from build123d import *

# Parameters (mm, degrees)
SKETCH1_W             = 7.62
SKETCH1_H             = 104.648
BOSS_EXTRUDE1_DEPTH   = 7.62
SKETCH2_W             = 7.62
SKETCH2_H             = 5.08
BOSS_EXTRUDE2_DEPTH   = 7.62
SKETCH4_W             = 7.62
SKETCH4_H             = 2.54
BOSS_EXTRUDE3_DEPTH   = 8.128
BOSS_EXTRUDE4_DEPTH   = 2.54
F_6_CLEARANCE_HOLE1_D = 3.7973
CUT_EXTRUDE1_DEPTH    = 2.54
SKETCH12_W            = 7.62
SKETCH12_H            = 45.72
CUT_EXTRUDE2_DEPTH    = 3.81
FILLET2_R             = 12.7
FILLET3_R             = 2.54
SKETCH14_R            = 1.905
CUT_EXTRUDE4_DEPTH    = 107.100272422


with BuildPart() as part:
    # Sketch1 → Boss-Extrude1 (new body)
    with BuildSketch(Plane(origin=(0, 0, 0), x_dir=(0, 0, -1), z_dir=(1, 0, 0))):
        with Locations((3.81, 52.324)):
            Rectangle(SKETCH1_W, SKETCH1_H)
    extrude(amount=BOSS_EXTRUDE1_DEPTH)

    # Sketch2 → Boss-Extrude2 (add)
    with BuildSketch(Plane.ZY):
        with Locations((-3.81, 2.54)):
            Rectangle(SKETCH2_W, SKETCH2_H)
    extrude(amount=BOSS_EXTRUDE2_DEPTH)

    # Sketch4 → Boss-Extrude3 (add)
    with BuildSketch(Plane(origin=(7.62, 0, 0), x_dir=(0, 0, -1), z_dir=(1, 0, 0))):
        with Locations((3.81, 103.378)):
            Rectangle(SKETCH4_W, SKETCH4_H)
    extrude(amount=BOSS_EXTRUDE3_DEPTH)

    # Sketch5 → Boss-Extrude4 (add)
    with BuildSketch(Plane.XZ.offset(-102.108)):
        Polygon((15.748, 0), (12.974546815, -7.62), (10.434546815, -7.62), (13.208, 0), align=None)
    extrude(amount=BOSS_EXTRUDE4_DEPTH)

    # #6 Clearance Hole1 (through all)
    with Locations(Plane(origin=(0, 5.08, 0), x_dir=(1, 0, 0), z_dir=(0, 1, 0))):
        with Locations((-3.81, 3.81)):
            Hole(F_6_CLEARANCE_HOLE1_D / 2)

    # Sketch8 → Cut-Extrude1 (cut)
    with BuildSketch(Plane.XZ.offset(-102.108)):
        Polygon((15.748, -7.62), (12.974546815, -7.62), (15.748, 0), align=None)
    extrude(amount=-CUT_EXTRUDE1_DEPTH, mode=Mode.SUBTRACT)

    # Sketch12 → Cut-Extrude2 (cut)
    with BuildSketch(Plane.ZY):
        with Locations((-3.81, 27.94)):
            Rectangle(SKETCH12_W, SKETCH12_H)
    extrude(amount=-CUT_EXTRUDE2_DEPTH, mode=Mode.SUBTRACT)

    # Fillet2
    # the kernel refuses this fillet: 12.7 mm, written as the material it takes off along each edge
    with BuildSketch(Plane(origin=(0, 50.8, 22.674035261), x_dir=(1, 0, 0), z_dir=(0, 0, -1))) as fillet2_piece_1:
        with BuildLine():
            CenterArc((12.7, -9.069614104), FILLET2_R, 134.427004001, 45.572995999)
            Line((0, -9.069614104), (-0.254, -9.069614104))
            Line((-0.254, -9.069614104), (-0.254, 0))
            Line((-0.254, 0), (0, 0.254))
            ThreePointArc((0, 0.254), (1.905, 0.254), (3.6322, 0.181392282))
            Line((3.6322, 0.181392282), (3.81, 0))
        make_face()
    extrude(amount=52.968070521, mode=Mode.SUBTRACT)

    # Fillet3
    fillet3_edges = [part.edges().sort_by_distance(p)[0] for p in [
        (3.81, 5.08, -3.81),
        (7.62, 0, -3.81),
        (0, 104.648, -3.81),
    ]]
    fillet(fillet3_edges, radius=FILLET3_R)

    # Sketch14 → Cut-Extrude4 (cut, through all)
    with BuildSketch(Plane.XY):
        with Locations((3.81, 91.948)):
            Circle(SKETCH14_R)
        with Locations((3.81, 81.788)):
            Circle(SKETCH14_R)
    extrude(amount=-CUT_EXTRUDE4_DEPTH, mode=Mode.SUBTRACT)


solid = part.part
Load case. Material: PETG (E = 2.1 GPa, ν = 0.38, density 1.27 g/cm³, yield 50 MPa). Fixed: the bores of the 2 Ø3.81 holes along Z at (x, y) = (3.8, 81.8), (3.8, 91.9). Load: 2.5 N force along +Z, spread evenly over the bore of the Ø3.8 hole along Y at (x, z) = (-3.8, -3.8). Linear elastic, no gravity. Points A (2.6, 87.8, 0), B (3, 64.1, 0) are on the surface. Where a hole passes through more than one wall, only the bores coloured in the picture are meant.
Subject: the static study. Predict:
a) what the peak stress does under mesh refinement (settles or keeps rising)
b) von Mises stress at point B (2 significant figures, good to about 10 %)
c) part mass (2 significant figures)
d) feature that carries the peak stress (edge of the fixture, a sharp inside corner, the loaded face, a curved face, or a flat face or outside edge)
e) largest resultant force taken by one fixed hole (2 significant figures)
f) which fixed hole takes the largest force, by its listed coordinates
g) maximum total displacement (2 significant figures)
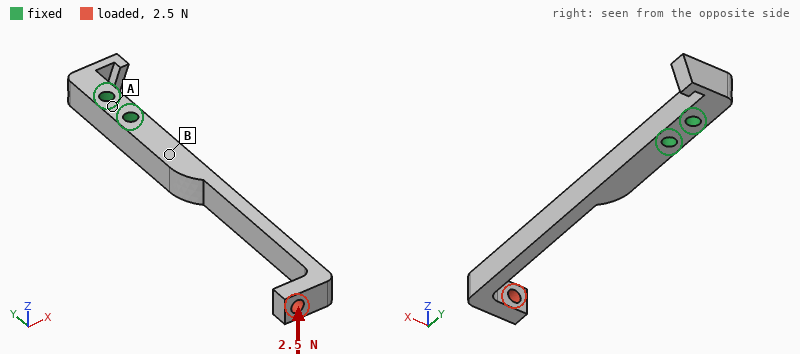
keeps rising
2.1 MPa
6.2 g
edge of the fixture
3.5 N
(3.8, 81.8)
1.2 mm
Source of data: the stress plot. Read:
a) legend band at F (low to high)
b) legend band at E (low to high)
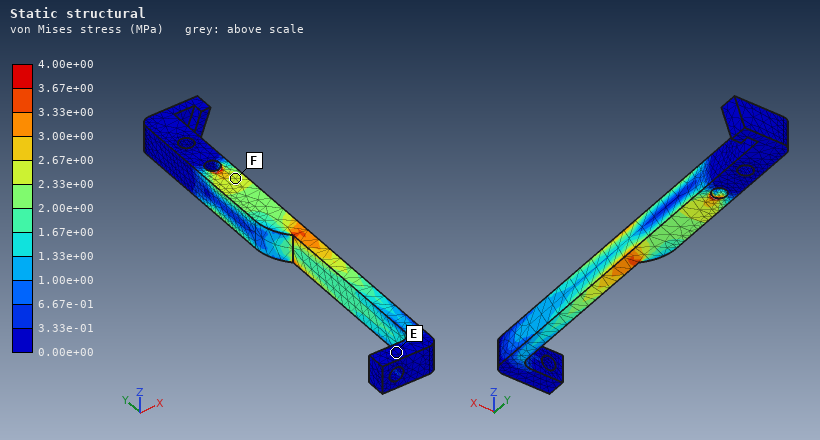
2.33e+00 to 2.67e+00 MPa
0.00e+00 to 3.33e-01 MPa
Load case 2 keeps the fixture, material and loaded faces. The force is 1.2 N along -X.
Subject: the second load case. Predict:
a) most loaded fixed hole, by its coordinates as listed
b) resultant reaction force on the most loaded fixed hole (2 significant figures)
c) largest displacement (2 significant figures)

(3.8, 81.8)
3.1 N
1.1 mm
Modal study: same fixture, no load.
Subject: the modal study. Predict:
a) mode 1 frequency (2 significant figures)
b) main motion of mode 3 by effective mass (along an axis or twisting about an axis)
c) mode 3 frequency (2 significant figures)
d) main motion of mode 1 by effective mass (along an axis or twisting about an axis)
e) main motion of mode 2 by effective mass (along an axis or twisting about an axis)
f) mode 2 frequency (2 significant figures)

170 Hz
along X
850 Hz
along X
along Z
240 Hz
